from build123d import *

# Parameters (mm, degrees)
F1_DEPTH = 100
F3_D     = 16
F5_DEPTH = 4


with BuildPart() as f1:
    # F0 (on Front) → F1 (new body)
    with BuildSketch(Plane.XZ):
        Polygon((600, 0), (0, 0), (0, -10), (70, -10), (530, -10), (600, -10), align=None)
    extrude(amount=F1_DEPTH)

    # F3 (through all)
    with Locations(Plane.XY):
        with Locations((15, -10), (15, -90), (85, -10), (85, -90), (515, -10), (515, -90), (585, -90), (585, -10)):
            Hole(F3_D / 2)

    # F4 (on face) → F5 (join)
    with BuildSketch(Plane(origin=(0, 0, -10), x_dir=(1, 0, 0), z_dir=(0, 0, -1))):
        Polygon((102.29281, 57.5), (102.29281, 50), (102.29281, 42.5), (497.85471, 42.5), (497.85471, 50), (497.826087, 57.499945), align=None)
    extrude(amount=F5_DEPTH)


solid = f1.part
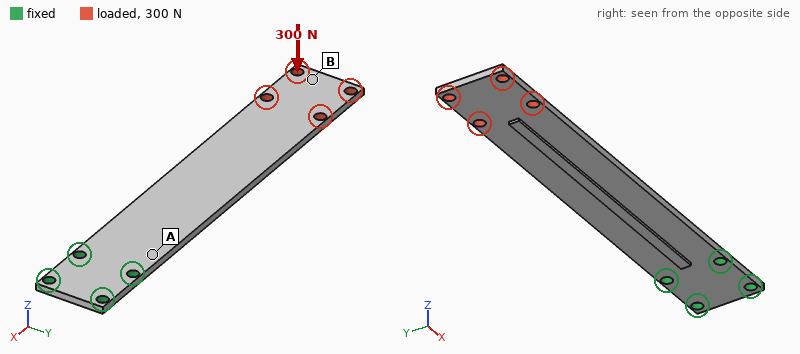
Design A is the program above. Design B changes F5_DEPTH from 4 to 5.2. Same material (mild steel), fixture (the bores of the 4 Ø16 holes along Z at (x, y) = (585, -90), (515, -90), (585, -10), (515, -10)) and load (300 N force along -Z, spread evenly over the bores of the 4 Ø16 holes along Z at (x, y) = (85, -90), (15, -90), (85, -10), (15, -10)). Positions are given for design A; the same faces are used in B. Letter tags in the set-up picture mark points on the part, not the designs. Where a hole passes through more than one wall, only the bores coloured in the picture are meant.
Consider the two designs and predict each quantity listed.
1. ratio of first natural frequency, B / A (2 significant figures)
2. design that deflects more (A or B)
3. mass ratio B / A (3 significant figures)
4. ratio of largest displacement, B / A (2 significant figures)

1.0
A
1.01
0.91
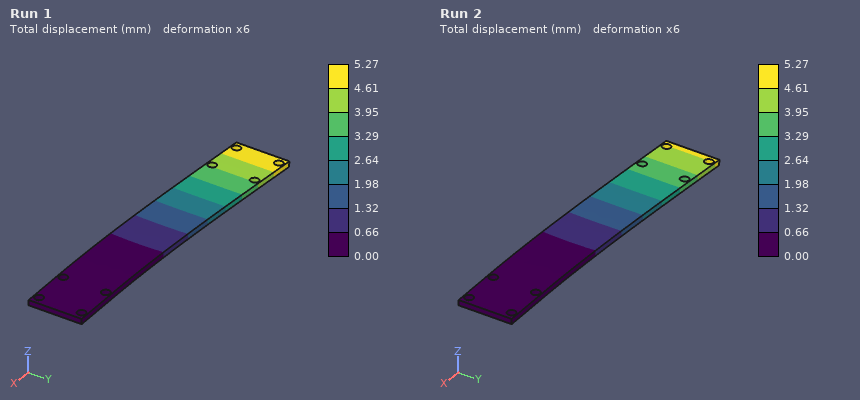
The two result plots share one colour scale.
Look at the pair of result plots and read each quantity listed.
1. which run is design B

Run 2
